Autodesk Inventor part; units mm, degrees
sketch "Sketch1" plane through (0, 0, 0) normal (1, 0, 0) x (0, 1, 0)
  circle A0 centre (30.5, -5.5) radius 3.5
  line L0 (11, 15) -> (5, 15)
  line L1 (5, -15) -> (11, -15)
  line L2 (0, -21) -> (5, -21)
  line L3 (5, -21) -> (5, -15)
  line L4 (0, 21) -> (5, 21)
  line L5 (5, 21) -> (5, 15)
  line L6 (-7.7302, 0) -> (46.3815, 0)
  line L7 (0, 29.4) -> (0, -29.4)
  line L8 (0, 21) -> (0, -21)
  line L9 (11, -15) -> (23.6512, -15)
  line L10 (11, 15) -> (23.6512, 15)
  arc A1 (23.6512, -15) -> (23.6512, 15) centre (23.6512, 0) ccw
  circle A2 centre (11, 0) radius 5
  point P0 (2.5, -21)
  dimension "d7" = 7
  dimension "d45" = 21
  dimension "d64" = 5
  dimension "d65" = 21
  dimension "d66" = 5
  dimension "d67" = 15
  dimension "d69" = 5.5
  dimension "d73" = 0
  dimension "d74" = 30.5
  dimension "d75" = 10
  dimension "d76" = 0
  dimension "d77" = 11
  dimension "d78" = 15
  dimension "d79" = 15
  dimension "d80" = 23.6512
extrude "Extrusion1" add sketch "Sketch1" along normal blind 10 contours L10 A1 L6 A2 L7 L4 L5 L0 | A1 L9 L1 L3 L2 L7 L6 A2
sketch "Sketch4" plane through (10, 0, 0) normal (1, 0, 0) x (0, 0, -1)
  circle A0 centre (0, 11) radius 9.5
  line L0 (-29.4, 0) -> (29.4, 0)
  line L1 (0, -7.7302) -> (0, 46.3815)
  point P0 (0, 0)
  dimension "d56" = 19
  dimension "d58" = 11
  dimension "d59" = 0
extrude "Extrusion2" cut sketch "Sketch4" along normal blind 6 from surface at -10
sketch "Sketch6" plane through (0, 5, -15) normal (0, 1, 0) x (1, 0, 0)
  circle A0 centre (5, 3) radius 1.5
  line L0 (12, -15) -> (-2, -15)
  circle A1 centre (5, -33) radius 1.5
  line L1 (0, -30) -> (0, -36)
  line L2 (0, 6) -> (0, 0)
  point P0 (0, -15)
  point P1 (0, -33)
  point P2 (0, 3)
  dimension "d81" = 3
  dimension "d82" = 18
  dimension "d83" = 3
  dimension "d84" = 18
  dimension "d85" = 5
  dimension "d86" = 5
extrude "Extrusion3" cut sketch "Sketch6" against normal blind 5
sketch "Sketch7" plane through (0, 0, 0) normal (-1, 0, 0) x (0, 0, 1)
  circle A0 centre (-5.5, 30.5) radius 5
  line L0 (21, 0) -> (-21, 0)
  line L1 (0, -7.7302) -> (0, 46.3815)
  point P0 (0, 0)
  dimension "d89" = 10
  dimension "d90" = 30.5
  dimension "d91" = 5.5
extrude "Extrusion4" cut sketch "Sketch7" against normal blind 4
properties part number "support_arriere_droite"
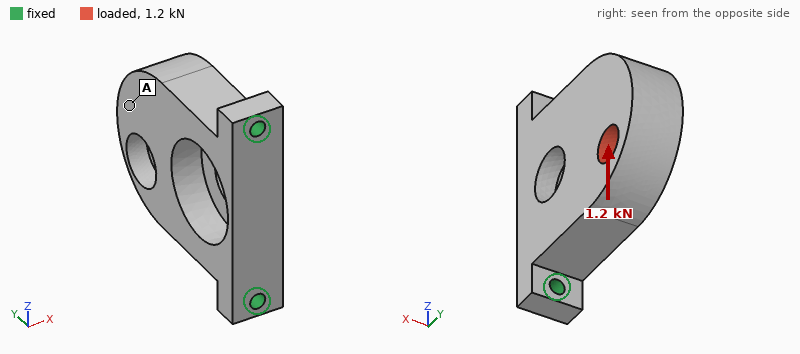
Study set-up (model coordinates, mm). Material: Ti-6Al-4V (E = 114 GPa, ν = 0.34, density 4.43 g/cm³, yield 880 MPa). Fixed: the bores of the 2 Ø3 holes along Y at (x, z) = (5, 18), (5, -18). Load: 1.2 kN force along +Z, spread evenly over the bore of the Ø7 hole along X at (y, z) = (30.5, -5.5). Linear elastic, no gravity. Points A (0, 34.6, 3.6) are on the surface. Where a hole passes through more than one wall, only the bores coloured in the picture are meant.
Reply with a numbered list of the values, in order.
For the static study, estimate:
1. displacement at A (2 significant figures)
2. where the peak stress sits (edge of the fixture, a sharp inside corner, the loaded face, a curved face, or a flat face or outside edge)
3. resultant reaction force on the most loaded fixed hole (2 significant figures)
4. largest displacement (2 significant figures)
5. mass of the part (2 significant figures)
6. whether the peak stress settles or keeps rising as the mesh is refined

1. 16 µm
2. edge of the fixture
3. 1.2 kN
4. 18 µm
5. 38 g
6. keeps rising
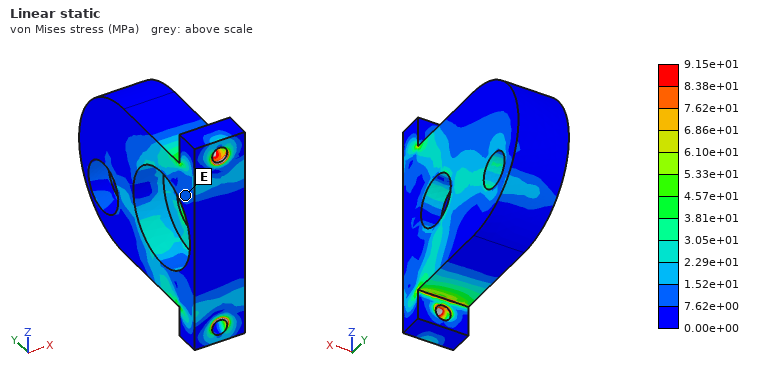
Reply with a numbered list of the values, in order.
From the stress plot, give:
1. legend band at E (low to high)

1. 7.62e+00 to 1.52e+01 MPa
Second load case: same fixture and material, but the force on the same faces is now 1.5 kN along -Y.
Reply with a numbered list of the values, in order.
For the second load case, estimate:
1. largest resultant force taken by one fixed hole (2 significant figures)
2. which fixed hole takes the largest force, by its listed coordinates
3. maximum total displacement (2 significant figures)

1. 1.0 kN
2. (5, -18)
3. 28 µm
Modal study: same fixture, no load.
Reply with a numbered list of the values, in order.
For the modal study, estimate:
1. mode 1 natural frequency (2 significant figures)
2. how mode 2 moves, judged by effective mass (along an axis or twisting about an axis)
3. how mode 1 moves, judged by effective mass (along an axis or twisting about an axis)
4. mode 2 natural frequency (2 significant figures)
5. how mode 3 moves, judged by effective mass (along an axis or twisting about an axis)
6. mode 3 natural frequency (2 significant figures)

1. 2900 Hz
2. along Z
3. along X
4. 9700 Hz
5. along Z
6. 12 kHz
